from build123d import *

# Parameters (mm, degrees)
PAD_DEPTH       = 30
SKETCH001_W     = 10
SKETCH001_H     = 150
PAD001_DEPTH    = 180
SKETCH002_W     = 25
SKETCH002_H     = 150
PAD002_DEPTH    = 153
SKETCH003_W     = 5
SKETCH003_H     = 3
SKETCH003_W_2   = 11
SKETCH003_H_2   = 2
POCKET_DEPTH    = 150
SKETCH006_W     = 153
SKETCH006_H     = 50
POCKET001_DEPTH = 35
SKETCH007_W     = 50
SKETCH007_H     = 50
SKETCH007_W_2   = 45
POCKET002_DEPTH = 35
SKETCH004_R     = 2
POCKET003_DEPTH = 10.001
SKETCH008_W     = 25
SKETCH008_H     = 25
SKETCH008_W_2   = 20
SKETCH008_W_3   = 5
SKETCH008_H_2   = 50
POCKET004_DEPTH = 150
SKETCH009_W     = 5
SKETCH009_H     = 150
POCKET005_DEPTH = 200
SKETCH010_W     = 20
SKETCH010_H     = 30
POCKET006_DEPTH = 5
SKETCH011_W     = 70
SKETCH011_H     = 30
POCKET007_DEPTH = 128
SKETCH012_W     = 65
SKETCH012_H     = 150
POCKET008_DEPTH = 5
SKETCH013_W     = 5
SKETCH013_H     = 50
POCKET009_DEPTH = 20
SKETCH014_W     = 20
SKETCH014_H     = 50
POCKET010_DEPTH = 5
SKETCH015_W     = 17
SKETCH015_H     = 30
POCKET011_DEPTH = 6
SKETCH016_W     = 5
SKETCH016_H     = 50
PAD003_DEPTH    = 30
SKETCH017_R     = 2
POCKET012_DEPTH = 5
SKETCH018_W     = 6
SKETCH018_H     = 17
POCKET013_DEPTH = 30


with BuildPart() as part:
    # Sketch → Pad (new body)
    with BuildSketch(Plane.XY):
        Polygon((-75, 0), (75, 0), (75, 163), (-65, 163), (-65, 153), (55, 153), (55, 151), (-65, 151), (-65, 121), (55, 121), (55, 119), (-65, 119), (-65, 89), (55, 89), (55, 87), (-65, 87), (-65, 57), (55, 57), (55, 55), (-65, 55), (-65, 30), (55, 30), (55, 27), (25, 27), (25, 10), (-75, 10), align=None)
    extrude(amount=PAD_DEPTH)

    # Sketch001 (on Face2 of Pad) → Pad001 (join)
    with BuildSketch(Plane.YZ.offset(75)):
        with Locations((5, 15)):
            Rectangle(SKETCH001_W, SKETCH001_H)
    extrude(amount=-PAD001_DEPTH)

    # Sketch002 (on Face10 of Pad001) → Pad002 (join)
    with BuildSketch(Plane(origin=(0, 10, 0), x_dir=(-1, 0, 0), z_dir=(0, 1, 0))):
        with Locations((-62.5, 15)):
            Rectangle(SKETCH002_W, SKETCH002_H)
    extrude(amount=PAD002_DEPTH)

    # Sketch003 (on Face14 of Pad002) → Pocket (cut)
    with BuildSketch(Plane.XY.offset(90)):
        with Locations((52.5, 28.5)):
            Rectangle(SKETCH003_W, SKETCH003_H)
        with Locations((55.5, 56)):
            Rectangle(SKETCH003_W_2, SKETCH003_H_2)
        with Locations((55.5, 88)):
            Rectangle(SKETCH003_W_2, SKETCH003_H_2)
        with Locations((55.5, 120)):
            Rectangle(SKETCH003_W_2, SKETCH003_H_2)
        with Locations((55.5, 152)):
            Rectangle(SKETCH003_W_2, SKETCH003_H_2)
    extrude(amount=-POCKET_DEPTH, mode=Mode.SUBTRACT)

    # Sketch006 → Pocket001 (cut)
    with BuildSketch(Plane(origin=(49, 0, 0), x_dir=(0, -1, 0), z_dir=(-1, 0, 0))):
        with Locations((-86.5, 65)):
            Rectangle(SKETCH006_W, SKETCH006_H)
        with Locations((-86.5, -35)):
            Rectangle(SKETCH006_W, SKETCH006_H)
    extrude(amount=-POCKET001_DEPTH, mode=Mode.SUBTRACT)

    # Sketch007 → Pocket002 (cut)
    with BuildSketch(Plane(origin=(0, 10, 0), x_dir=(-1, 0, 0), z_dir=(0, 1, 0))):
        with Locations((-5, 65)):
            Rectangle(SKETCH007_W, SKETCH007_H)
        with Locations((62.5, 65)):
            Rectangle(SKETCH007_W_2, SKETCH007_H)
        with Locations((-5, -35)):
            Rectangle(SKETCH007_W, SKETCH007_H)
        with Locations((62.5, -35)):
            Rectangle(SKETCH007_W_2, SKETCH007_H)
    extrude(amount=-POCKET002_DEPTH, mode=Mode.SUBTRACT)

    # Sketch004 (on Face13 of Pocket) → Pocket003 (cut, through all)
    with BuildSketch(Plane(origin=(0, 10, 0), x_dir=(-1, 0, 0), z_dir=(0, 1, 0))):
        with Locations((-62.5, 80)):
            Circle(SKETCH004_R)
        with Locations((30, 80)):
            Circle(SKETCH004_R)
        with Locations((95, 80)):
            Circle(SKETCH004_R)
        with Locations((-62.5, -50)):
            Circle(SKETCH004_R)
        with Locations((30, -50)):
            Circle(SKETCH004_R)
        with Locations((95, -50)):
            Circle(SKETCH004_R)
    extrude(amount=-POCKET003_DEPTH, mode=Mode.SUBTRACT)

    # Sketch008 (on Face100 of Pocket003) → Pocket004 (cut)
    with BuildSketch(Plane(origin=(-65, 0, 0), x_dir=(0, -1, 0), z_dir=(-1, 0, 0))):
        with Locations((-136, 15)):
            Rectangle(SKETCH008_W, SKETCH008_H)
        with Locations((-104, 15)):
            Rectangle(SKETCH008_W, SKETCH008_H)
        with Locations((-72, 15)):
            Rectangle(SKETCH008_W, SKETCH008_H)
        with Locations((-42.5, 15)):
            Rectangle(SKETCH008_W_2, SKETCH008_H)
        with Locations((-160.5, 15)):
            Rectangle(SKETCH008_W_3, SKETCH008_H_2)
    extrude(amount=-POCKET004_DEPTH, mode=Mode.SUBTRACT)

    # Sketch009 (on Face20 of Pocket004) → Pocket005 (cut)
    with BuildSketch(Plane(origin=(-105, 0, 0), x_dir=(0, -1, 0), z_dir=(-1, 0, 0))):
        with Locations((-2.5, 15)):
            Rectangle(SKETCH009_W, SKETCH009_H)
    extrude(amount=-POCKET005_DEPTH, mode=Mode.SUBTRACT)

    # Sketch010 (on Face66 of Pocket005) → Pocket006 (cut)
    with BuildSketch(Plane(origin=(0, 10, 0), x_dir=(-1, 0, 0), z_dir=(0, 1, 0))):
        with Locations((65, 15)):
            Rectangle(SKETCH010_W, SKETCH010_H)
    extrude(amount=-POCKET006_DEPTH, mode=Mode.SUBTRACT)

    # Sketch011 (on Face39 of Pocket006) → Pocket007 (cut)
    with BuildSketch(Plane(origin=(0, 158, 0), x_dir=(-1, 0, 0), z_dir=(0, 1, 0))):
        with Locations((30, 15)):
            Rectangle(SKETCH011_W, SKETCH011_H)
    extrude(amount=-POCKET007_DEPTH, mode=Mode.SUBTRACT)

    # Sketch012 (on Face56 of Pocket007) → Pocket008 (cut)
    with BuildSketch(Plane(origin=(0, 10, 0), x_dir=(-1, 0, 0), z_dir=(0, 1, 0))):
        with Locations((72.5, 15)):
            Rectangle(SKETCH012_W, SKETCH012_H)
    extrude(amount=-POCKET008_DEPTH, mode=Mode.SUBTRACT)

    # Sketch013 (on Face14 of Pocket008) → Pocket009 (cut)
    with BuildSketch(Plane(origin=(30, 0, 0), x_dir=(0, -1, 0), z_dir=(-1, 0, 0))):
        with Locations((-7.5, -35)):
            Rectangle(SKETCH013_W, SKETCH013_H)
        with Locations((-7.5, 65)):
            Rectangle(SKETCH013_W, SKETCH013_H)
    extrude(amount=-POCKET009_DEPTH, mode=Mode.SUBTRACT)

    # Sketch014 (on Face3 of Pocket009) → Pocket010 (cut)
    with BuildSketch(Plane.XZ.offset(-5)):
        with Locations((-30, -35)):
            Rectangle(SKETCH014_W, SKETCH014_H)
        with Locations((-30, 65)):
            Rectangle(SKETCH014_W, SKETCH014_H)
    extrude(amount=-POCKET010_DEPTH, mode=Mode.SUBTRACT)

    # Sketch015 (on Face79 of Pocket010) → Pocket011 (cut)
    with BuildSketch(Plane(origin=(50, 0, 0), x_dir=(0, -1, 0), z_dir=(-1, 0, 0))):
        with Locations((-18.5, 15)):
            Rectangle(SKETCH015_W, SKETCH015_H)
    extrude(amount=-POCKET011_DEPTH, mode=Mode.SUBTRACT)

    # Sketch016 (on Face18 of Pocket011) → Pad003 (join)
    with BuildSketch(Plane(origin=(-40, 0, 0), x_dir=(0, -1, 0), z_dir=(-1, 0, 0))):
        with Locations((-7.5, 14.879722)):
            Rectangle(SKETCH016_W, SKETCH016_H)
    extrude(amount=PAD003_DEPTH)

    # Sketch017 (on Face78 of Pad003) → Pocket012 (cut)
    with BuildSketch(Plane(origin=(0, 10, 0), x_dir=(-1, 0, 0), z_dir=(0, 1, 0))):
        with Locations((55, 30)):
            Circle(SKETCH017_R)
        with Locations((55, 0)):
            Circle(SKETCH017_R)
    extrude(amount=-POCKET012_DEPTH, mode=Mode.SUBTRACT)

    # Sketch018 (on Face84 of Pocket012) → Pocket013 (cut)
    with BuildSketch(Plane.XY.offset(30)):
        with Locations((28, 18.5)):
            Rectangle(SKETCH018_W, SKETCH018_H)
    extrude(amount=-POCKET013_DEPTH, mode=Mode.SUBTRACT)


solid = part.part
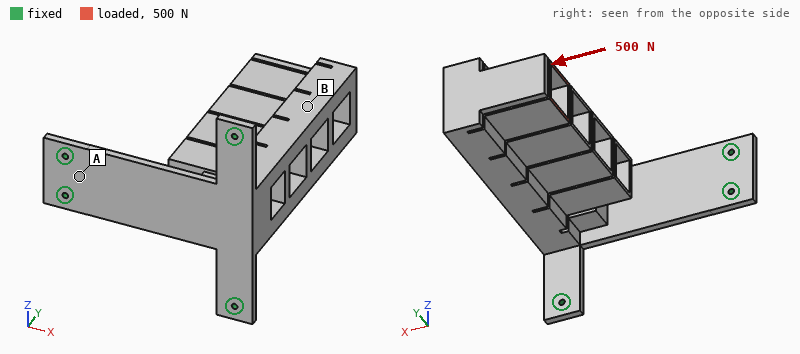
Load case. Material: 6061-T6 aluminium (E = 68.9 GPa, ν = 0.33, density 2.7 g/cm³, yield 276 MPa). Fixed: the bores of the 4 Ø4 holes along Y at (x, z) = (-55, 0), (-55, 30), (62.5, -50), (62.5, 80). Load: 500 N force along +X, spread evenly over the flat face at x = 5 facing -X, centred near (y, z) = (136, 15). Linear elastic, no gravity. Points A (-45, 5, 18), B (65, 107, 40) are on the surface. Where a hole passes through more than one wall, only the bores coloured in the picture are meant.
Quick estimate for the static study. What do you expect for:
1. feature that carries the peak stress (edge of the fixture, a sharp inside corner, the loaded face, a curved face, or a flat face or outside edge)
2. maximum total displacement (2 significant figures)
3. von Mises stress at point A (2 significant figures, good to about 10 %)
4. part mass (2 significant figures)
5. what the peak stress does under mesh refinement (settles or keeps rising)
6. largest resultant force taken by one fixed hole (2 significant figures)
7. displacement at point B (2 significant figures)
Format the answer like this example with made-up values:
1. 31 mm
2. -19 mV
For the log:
1. edge of the fixture
2. 2.7 mm
3. 52 MPa
4. 620 g
5. keeps rising
6. 420 N
7. 1.6 mm
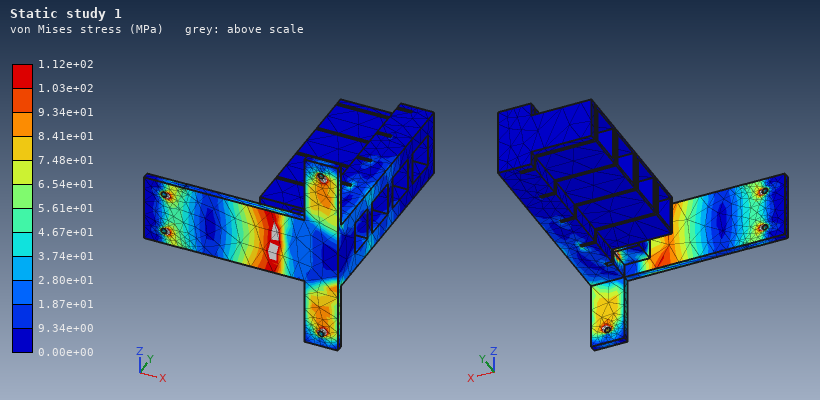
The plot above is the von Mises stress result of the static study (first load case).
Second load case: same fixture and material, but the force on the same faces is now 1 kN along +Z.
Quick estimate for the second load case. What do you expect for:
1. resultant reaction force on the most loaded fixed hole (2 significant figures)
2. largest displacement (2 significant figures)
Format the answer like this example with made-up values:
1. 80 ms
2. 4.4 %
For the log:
1. 1.3 kN
2. 2.1 mm
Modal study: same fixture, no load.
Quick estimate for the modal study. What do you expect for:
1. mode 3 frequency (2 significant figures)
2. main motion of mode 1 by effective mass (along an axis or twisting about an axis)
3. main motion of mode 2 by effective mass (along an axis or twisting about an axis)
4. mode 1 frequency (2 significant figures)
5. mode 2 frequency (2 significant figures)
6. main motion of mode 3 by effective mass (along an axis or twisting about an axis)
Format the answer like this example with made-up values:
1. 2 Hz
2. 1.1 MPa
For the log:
1. 510 Hz
2. along X
3. along Z
4. 160 Hz
5. 260 Hz
6. along Y
